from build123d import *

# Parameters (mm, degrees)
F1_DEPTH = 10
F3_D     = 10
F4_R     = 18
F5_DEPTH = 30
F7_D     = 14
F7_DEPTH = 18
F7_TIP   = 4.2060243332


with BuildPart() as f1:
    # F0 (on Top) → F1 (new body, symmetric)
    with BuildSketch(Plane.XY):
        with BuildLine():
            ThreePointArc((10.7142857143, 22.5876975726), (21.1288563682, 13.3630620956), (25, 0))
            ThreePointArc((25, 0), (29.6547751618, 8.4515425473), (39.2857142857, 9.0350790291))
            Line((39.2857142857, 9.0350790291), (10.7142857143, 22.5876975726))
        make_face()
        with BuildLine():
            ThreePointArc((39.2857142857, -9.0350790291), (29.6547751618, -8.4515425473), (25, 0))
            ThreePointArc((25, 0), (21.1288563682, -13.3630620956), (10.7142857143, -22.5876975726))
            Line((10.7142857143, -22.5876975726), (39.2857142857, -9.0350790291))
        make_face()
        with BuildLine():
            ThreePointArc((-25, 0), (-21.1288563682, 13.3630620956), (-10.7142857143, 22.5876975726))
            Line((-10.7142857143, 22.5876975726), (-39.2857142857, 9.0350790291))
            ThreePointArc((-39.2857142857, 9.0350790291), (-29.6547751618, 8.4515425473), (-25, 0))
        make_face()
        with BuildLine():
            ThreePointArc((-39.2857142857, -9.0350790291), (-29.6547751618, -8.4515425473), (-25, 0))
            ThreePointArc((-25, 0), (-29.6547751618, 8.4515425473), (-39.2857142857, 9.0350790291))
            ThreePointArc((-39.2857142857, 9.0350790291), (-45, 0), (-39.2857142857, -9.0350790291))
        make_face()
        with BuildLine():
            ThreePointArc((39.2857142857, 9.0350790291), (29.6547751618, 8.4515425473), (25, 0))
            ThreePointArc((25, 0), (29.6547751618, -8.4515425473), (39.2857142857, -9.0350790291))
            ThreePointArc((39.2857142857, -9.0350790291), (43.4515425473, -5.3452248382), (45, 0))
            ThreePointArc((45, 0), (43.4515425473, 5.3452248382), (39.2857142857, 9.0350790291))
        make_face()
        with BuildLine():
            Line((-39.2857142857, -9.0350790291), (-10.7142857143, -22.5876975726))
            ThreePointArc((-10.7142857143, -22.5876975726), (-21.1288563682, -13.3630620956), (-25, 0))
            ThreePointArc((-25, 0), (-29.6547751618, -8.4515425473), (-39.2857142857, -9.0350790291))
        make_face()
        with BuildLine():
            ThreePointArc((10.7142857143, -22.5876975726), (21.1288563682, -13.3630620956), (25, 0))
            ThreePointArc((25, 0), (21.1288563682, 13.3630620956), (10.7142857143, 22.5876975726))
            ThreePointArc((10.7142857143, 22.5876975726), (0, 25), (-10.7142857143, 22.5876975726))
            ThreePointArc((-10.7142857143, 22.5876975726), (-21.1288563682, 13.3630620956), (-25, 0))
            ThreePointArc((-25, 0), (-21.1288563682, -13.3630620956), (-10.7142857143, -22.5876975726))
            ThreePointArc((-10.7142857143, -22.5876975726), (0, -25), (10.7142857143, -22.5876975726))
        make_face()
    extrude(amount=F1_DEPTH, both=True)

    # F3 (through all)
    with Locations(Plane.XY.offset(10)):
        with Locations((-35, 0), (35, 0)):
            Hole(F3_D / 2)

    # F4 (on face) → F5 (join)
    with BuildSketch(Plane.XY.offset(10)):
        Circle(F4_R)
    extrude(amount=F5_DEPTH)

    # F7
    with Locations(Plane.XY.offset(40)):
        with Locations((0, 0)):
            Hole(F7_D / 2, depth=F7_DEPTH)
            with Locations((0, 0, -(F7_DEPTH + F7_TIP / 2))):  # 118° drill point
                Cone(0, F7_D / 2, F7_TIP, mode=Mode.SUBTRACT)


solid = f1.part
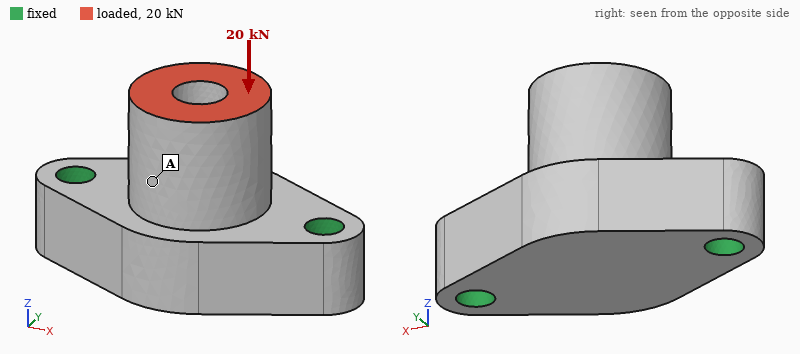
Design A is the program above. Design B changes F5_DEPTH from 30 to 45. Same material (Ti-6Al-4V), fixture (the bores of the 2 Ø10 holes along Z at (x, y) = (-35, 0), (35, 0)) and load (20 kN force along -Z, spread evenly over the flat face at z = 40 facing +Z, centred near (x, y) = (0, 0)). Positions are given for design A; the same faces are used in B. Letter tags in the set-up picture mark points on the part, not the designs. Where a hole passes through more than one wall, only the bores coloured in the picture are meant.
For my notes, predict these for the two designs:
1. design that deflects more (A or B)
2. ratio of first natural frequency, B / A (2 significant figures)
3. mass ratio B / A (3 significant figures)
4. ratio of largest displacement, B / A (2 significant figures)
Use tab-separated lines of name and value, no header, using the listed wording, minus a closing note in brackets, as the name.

design that deflects more	B
ratio of first natural frequency, B / A	0.67
mass ratio B / A	1.15
ratio of largest displacement, B / A	1.1
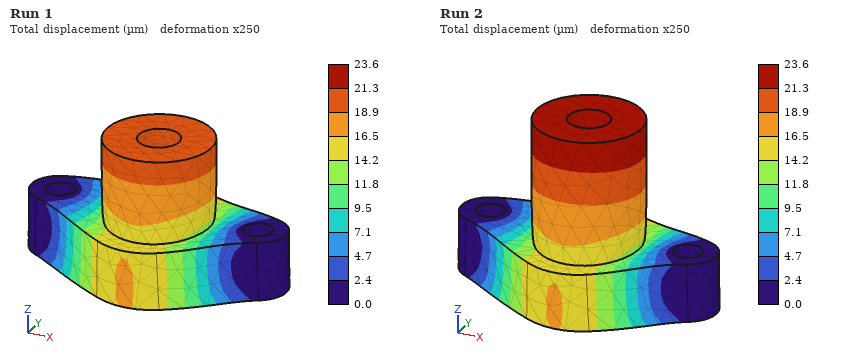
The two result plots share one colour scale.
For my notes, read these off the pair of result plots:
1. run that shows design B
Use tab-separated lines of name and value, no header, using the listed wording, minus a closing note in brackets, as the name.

run that shows design B	Run 2
